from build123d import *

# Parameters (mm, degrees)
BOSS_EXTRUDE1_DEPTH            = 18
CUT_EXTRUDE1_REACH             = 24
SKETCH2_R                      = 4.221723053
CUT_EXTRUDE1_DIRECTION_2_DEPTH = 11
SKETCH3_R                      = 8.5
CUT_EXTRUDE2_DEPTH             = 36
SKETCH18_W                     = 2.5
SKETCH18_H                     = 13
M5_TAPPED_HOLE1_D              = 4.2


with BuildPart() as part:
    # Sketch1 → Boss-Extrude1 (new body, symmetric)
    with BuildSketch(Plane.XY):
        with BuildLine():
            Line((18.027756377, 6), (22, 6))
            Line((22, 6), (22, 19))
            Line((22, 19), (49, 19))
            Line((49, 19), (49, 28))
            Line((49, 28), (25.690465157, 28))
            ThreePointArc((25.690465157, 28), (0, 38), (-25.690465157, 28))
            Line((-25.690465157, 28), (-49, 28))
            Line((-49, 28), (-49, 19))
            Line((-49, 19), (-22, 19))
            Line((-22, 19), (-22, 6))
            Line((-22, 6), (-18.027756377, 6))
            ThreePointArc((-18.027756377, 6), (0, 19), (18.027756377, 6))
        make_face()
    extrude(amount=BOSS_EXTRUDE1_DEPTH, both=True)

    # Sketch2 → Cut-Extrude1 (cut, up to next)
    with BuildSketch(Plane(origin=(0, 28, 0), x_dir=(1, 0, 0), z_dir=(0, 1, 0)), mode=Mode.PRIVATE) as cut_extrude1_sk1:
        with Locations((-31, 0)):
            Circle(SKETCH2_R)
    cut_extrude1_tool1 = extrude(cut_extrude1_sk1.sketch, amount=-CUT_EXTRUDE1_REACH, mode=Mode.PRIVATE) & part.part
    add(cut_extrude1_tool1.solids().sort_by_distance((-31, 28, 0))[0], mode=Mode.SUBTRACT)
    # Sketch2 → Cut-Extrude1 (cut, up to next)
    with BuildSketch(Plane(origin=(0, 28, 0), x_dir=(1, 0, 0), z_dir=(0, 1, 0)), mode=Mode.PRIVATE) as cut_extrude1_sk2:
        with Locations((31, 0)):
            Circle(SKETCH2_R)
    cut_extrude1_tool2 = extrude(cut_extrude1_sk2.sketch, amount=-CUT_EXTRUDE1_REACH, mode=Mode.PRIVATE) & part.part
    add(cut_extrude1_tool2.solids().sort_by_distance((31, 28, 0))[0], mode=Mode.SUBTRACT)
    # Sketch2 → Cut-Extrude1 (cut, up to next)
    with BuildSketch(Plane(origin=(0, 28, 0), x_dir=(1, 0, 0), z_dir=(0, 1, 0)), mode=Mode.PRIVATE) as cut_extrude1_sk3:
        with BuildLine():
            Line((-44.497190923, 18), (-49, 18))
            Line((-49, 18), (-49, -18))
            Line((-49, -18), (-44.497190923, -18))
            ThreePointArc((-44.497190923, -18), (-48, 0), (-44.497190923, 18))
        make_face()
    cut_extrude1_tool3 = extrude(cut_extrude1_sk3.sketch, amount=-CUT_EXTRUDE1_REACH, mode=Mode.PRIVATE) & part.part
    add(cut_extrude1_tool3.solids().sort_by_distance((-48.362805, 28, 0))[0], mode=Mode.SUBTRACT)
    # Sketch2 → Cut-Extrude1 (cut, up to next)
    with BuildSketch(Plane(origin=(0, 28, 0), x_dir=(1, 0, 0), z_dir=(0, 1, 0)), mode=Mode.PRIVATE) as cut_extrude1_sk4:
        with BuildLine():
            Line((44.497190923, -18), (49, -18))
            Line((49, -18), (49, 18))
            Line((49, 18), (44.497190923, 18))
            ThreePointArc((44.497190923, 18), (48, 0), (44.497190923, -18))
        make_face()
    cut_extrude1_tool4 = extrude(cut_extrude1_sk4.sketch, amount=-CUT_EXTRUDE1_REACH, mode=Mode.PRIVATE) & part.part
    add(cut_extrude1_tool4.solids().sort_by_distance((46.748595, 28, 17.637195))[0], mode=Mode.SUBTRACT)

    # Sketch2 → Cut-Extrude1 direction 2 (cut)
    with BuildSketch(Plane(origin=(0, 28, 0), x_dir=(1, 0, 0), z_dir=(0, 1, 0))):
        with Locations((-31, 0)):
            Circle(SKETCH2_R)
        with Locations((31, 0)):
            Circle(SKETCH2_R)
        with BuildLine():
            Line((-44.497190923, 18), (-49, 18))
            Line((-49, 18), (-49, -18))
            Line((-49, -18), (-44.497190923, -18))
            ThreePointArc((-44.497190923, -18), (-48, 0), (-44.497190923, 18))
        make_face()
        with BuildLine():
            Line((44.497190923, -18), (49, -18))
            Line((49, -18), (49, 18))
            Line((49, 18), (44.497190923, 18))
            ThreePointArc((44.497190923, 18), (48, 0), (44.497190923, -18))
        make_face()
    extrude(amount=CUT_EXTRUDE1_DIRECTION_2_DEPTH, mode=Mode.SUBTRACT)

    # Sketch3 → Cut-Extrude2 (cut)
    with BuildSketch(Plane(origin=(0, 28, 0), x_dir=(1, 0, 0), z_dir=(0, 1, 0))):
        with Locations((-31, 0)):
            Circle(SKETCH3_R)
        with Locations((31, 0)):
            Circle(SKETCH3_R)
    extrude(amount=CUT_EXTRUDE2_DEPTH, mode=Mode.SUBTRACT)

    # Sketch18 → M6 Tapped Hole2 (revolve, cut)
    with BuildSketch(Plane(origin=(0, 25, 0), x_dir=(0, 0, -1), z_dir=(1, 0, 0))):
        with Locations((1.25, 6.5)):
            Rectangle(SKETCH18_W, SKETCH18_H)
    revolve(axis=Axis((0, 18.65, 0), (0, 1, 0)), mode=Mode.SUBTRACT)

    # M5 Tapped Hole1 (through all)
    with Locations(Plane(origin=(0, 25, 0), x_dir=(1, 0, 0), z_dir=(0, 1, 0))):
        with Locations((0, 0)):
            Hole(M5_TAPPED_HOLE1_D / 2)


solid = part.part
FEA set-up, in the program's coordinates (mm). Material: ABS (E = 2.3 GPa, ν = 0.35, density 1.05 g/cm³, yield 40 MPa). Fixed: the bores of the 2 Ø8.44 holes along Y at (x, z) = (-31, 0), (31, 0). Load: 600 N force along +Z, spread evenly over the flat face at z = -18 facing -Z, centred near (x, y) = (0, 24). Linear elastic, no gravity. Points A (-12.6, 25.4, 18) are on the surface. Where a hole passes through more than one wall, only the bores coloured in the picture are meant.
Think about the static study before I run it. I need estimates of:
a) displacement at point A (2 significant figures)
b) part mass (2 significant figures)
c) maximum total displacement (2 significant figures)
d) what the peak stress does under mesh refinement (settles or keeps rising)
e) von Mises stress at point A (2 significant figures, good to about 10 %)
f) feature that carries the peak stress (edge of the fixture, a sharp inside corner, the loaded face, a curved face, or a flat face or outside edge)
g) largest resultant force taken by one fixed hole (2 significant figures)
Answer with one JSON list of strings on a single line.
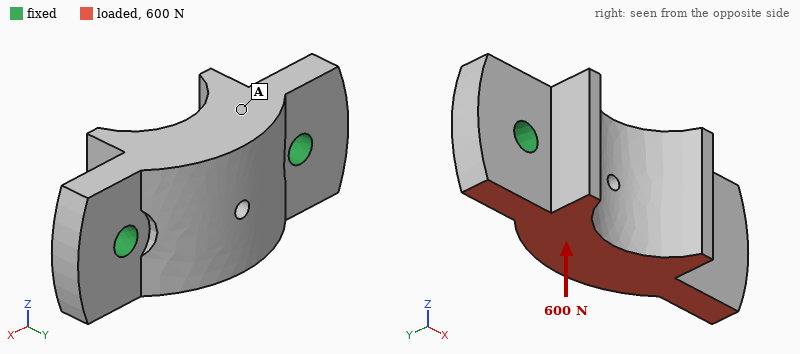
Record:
["16 µm", "52 g", "28 µm", "keeps rising", "0.83 MPa", "edge of the fixture", "300 N"]
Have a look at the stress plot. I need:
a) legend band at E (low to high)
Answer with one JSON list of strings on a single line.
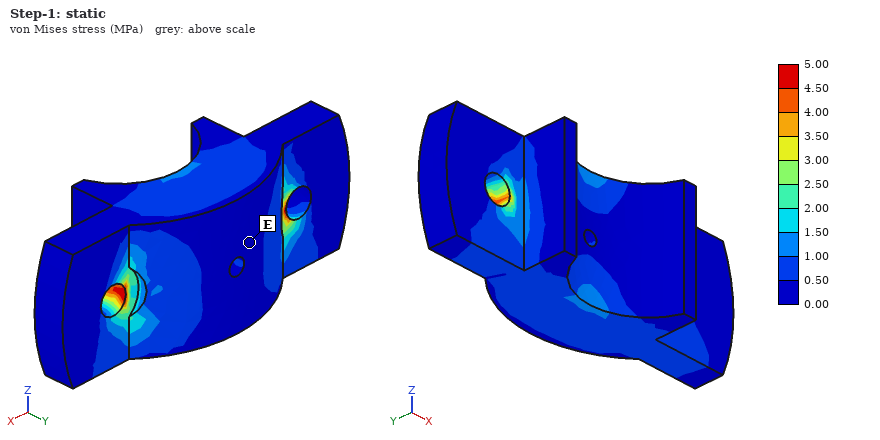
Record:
["0.00 to 0.50 MPa"]
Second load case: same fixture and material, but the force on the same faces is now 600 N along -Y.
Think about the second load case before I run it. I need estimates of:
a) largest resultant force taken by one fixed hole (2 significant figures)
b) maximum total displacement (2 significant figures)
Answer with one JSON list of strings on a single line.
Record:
["310 N", "0.17 mm"]
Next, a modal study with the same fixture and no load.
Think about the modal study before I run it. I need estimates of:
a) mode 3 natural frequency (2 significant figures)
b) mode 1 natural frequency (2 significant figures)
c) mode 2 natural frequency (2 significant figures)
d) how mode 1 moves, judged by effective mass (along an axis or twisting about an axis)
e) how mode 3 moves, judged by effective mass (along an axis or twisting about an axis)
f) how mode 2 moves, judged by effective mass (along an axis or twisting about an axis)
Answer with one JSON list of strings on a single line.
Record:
["4200 Hz", "2500 Hz", "3300 Hz", "twisting about X", "along Z", "along Y"]
